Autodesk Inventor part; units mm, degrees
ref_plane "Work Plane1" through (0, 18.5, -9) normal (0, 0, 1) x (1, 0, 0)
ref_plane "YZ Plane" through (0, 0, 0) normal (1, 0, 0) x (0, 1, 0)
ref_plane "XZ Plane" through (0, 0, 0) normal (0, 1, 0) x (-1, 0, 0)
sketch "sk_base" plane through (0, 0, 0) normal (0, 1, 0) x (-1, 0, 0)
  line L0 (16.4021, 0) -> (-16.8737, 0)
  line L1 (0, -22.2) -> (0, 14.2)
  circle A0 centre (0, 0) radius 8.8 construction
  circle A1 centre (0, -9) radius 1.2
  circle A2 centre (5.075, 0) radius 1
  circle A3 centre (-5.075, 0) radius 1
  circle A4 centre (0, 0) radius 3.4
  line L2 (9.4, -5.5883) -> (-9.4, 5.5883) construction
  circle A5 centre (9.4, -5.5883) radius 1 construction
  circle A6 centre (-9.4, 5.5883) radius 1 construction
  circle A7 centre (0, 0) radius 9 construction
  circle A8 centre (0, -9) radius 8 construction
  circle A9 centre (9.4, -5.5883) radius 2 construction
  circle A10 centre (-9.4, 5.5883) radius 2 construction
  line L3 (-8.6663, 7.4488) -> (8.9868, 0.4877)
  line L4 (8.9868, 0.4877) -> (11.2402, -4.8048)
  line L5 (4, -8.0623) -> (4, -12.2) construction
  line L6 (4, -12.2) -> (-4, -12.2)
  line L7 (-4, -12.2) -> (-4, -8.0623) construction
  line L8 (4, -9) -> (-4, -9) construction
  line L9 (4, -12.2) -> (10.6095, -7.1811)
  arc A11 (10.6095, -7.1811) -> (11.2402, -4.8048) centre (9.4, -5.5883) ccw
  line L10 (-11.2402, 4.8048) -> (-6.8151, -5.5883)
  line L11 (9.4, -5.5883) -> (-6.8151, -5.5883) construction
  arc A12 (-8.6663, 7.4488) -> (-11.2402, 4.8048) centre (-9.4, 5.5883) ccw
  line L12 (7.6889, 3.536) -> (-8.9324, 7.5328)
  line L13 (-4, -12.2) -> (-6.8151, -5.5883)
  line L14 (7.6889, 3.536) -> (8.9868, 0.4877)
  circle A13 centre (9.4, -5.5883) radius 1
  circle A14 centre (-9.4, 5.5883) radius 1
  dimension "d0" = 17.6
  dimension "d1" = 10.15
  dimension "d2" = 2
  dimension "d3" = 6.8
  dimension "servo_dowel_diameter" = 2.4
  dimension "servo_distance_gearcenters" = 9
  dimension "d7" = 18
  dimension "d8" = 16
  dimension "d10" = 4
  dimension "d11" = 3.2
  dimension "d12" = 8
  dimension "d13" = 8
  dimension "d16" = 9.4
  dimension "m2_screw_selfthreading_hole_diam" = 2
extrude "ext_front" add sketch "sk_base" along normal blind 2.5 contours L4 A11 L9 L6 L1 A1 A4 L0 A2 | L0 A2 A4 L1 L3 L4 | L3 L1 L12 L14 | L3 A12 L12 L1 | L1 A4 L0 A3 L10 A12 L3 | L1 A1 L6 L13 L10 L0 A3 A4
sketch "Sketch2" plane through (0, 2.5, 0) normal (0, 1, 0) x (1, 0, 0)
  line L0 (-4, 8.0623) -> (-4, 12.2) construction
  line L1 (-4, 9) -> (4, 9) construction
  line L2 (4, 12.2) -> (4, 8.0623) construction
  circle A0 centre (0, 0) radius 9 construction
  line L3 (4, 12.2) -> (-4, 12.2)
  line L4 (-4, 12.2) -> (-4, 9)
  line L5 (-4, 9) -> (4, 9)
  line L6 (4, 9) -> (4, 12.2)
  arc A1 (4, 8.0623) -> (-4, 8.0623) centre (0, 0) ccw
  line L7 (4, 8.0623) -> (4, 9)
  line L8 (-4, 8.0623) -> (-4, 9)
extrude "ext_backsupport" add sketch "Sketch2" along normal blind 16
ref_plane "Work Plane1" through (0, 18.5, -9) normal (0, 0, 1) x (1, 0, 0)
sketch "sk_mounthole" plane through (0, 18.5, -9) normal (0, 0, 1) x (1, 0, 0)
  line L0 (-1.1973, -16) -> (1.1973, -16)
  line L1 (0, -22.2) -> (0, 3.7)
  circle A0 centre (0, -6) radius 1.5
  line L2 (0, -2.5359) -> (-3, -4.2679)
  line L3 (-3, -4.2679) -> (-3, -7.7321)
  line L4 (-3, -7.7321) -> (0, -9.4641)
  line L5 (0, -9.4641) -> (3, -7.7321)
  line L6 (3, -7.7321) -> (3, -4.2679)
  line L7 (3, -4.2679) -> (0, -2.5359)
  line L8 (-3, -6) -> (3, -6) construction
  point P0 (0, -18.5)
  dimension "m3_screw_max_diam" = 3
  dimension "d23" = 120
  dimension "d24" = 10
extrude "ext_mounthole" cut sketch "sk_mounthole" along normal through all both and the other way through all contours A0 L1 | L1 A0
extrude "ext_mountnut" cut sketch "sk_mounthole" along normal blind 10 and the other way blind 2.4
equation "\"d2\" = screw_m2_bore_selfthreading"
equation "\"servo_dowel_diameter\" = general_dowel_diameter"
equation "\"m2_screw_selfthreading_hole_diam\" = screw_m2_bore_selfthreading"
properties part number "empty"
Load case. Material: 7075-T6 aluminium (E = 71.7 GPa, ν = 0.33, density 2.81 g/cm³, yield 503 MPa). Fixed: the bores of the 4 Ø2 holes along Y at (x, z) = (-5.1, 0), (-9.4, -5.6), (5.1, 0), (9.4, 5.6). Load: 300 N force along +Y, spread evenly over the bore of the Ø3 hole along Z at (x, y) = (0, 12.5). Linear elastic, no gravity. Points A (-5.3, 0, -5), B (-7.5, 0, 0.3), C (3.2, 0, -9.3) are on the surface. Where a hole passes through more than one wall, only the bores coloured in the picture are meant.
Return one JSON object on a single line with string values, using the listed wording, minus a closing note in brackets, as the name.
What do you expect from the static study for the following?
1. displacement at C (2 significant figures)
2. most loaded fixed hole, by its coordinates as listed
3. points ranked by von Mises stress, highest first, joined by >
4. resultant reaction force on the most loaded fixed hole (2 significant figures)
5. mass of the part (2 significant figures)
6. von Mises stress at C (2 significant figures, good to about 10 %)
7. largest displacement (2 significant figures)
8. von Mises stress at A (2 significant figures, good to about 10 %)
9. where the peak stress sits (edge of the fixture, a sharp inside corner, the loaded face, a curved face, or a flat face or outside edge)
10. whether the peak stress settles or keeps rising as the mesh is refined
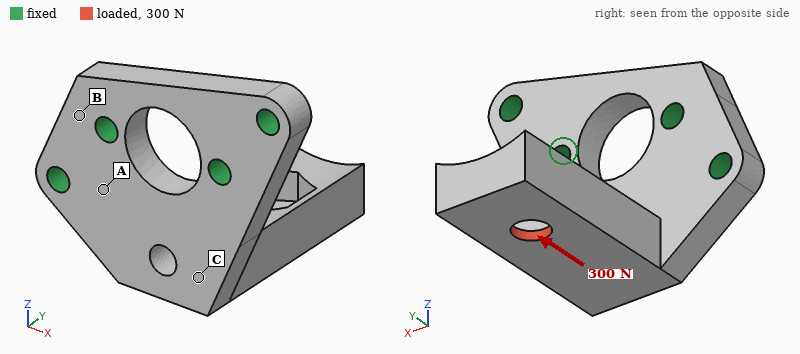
{"displacement at C": "0.063 mm", "most loaded fixed hole, by its coordinates as listed": "(-9.4, -5.6)", "points ranked by von Mises stress, highest first, joined by >": "A > C > B", "resultant reaction force on the most loaded fixed hole": "240 N", "mass of the part": "2.8 g", "von Mises stress at C": "62 MPa", "largest displacement": "0.24 mm", "von Mises stress at A": "110 MPa", "where the peak stress sits": "edge of the fixture", "whether the peak stress settles or keeps rising as the mesh is refined": "keeps rising"}
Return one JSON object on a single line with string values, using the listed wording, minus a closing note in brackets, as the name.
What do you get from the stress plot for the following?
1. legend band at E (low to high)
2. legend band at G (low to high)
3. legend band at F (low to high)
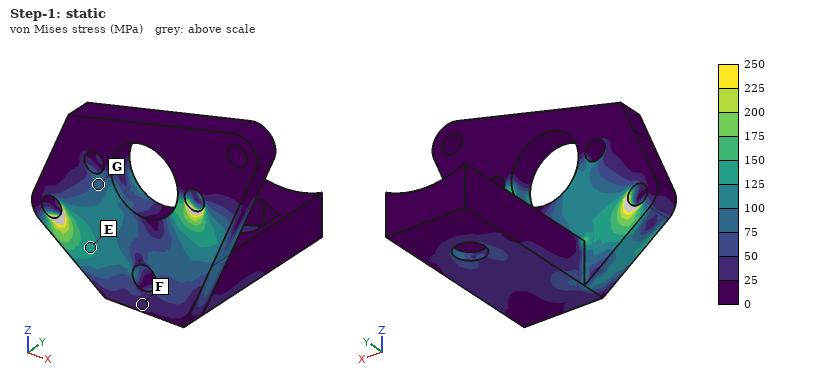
{"legend band at E": "125 to 150 MPa", "legend band at G": "75 to 100 MPa", "legend band at F": "25 to 50 MPa"}
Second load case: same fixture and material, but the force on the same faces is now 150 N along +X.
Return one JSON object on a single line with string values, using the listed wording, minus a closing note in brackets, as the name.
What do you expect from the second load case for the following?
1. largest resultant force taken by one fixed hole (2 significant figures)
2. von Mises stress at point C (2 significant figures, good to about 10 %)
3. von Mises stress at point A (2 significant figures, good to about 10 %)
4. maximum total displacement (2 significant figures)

{"largest resultant force taken by one fixed hole": "160 N", "von Mises stress at point C": "60 MPa", "von Mises stress at point A": "23 MPa", "maximum total displacement": "97 µm"}
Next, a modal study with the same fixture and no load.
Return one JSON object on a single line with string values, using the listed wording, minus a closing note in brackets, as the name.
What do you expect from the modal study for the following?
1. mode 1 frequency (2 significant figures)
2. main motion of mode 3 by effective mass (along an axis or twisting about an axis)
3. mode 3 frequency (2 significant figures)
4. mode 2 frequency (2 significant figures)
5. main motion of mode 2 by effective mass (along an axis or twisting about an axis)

{"mode 1 frequency": "5000 Hz", "main motion of mode 3 by effective mass": "along Y", "mode 3 frequency": "17 kHz", "mode 2 frequency": "9000 Hz", "main motion of mode 2 by effective mass": "along X"}
